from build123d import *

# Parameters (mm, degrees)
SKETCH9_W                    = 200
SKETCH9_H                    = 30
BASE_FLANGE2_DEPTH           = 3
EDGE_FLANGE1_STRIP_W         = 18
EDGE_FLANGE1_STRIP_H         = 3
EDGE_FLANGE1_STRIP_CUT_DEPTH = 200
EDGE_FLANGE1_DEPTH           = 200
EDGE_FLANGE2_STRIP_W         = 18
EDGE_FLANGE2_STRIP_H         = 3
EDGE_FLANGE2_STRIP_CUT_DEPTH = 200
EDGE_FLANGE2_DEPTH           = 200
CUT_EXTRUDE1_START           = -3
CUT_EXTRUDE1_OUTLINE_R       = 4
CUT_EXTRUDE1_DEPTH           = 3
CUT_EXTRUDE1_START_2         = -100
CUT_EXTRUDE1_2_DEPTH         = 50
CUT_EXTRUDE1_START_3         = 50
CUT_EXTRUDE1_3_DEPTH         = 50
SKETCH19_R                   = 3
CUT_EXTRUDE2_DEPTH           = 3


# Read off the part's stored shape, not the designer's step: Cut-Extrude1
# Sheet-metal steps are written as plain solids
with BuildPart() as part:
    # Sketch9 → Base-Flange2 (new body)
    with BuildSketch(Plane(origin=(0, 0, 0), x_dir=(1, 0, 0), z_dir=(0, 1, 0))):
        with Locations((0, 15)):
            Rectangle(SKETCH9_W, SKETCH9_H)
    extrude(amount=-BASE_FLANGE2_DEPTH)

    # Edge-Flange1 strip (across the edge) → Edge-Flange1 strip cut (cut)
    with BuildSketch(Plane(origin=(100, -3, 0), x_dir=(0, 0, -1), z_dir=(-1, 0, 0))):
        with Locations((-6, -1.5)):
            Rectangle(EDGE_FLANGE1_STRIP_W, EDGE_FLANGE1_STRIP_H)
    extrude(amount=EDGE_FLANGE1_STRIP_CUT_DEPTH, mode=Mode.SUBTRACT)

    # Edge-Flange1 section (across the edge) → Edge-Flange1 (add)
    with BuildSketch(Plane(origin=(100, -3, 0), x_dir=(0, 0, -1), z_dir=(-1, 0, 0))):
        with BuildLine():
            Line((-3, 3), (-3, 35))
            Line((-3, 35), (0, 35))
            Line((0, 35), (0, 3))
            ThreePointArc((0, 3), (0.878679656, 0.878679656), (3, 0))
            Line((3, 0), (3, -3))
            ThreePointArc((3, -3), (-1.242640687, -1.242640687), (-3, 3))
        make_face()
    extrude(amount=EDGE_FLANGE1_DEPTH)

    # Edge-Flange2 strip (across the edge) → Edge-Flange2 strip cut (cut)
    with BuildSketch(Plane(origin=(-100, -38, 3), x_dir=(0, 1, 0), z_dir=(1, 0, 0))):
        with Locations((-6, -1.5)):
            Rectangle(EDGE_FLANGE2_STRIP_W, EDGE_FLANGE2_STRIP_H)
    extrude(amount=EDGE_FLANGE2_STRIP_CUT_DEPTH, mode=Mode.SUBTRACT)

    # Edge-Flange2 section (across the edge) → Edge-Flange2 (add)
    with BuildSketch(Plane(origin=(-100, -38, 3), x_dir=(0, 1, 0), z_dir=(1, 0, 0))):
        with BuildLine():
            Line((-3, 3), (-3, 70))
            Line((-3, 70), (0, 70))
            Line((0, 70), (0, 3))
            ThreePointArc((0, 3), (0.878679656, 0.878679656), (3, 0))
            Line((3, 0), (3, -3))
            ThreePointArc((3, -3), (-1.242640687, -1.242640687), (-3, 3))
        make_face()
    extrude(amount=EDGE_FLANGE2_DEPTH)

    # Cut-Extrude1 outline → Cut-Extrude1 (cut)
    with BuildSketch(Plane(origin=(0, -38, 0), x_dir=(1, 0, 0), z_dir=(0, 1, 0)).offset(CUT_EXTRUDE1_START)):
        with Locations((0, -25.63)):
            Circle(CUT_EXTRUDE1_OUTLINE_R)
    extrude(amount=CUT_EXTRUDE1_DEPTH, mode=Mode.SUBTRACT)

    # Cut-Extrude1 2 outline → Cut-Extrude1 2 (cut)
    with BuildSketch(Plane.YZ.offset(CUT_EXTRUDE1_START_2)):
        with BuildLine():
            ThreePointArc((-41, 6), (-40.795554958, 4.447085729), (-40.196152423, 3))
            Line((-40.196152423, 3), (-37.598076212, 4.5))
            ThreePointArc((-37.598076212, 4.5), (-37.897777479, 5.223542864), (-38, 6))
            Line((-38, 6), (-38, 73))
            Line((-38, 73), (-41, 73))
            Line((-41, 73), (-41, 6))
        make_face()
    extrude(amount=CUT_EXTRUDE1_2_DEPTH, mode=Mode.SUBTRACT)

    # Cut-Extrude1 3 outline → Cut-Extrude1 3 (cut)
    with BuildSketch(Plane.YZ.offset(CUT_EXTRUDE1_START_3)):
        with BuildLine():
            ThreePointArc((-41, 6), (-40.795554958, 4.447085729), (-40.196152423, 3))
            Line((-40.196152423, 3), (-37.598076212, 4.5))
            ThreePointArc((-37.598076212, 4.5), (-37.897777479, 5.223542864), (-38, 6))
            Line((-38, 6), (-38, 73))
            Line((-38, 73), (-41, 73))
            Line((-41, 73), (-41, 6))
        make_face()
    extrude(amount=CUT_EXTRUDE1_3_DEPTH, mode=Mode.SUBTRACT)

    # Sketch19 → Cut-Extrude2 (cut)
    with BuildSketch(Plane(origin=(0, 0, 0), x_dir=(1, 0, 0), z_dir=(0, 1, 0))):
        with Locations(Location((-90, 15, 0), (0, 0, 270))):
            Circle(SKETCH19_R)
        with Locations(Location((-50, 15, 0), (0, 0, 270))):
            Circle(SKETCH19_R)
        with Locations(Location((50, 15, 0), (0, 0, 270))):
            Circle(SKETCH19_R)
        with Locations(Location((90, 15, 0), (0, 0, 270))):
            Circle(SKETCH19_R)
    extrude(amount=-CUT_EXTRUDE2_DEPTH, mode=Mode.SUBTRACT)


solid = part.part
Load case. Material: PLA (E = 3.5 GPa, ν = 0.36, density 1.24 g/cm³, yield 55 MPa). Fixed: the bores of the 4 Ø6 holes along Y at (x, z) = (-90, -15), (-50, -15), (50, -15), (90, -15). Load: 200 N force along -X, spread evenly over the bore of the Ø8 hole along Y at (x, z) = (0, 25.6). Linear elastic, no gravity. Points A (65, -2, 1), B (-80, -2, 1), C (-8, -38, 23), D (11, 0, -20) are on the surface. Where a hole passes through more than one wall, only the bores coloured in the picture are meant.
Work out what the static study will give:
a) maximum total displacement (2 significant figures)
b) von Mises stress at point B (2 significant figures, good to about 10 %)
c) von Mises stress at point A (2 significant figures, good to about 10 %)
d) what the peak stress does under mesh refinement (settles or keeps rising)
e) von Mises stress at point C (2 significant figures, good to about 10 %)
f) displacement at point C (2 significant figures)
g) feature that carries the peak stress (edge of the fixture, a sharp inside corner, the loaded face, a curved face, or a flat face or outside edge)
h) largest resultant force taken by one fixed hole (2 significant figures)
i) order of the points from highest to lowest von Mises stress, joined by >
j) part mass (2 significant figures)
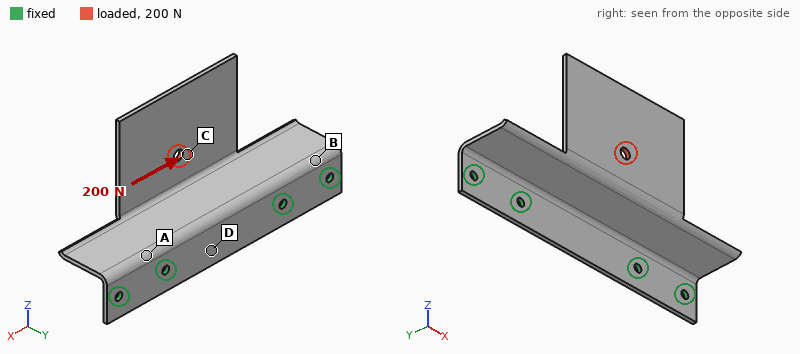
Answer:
2.6 mm
5.8 MPa
7.0 MPa
keeps rising
4.3 MPa
0.63 mm
a sharp inside corner
99 N
A > B > C > D
76 g
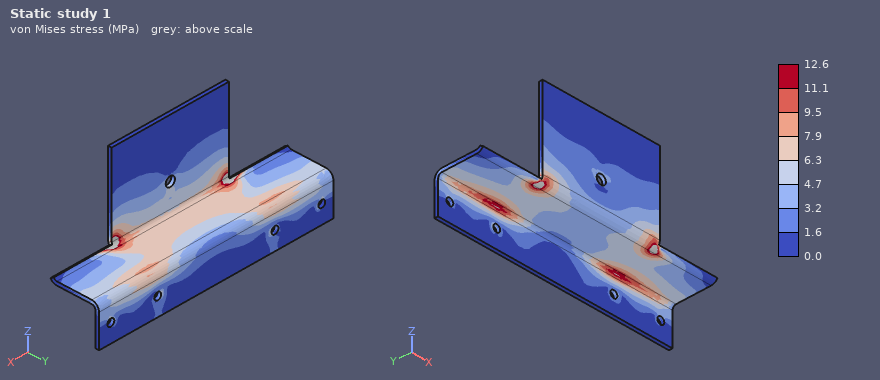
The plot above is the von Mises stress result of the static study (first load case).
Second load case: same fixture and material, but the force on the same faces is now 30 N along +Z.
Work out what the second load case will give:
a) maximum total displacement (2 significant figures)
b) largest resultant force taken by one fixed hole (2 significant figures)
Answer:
2.3 mm
24 N
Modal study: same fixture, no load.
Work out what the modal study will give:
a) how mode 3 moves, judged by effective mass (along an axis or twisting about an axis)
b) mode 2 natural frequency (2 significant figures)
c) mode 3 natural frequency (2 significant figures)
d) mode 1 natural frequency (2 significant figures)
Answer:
along Z
200 Hz
250 Hz
85 Hz
